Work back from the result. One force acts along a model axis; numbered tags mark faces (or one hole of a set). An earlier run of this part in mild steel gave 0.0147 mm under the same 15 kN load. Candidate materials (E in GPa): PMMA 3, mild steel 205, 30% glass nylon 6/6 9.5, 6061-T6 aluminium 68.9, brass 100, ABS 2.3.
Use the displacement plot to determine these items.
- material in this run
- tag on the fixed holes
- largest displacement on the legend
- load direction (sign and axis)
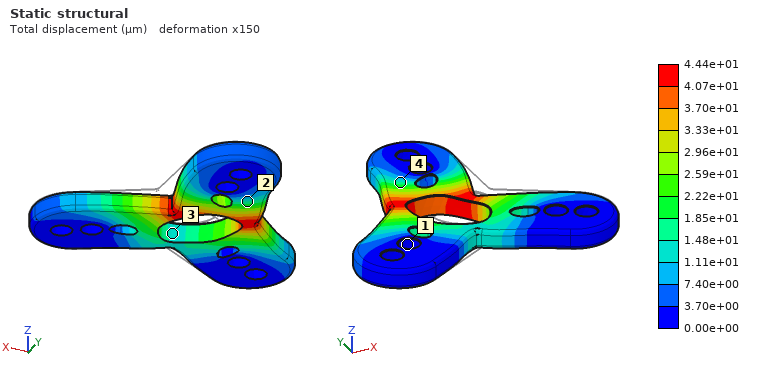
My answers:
6061-T6 aluminium
1
4.44e+01 µm
-X
